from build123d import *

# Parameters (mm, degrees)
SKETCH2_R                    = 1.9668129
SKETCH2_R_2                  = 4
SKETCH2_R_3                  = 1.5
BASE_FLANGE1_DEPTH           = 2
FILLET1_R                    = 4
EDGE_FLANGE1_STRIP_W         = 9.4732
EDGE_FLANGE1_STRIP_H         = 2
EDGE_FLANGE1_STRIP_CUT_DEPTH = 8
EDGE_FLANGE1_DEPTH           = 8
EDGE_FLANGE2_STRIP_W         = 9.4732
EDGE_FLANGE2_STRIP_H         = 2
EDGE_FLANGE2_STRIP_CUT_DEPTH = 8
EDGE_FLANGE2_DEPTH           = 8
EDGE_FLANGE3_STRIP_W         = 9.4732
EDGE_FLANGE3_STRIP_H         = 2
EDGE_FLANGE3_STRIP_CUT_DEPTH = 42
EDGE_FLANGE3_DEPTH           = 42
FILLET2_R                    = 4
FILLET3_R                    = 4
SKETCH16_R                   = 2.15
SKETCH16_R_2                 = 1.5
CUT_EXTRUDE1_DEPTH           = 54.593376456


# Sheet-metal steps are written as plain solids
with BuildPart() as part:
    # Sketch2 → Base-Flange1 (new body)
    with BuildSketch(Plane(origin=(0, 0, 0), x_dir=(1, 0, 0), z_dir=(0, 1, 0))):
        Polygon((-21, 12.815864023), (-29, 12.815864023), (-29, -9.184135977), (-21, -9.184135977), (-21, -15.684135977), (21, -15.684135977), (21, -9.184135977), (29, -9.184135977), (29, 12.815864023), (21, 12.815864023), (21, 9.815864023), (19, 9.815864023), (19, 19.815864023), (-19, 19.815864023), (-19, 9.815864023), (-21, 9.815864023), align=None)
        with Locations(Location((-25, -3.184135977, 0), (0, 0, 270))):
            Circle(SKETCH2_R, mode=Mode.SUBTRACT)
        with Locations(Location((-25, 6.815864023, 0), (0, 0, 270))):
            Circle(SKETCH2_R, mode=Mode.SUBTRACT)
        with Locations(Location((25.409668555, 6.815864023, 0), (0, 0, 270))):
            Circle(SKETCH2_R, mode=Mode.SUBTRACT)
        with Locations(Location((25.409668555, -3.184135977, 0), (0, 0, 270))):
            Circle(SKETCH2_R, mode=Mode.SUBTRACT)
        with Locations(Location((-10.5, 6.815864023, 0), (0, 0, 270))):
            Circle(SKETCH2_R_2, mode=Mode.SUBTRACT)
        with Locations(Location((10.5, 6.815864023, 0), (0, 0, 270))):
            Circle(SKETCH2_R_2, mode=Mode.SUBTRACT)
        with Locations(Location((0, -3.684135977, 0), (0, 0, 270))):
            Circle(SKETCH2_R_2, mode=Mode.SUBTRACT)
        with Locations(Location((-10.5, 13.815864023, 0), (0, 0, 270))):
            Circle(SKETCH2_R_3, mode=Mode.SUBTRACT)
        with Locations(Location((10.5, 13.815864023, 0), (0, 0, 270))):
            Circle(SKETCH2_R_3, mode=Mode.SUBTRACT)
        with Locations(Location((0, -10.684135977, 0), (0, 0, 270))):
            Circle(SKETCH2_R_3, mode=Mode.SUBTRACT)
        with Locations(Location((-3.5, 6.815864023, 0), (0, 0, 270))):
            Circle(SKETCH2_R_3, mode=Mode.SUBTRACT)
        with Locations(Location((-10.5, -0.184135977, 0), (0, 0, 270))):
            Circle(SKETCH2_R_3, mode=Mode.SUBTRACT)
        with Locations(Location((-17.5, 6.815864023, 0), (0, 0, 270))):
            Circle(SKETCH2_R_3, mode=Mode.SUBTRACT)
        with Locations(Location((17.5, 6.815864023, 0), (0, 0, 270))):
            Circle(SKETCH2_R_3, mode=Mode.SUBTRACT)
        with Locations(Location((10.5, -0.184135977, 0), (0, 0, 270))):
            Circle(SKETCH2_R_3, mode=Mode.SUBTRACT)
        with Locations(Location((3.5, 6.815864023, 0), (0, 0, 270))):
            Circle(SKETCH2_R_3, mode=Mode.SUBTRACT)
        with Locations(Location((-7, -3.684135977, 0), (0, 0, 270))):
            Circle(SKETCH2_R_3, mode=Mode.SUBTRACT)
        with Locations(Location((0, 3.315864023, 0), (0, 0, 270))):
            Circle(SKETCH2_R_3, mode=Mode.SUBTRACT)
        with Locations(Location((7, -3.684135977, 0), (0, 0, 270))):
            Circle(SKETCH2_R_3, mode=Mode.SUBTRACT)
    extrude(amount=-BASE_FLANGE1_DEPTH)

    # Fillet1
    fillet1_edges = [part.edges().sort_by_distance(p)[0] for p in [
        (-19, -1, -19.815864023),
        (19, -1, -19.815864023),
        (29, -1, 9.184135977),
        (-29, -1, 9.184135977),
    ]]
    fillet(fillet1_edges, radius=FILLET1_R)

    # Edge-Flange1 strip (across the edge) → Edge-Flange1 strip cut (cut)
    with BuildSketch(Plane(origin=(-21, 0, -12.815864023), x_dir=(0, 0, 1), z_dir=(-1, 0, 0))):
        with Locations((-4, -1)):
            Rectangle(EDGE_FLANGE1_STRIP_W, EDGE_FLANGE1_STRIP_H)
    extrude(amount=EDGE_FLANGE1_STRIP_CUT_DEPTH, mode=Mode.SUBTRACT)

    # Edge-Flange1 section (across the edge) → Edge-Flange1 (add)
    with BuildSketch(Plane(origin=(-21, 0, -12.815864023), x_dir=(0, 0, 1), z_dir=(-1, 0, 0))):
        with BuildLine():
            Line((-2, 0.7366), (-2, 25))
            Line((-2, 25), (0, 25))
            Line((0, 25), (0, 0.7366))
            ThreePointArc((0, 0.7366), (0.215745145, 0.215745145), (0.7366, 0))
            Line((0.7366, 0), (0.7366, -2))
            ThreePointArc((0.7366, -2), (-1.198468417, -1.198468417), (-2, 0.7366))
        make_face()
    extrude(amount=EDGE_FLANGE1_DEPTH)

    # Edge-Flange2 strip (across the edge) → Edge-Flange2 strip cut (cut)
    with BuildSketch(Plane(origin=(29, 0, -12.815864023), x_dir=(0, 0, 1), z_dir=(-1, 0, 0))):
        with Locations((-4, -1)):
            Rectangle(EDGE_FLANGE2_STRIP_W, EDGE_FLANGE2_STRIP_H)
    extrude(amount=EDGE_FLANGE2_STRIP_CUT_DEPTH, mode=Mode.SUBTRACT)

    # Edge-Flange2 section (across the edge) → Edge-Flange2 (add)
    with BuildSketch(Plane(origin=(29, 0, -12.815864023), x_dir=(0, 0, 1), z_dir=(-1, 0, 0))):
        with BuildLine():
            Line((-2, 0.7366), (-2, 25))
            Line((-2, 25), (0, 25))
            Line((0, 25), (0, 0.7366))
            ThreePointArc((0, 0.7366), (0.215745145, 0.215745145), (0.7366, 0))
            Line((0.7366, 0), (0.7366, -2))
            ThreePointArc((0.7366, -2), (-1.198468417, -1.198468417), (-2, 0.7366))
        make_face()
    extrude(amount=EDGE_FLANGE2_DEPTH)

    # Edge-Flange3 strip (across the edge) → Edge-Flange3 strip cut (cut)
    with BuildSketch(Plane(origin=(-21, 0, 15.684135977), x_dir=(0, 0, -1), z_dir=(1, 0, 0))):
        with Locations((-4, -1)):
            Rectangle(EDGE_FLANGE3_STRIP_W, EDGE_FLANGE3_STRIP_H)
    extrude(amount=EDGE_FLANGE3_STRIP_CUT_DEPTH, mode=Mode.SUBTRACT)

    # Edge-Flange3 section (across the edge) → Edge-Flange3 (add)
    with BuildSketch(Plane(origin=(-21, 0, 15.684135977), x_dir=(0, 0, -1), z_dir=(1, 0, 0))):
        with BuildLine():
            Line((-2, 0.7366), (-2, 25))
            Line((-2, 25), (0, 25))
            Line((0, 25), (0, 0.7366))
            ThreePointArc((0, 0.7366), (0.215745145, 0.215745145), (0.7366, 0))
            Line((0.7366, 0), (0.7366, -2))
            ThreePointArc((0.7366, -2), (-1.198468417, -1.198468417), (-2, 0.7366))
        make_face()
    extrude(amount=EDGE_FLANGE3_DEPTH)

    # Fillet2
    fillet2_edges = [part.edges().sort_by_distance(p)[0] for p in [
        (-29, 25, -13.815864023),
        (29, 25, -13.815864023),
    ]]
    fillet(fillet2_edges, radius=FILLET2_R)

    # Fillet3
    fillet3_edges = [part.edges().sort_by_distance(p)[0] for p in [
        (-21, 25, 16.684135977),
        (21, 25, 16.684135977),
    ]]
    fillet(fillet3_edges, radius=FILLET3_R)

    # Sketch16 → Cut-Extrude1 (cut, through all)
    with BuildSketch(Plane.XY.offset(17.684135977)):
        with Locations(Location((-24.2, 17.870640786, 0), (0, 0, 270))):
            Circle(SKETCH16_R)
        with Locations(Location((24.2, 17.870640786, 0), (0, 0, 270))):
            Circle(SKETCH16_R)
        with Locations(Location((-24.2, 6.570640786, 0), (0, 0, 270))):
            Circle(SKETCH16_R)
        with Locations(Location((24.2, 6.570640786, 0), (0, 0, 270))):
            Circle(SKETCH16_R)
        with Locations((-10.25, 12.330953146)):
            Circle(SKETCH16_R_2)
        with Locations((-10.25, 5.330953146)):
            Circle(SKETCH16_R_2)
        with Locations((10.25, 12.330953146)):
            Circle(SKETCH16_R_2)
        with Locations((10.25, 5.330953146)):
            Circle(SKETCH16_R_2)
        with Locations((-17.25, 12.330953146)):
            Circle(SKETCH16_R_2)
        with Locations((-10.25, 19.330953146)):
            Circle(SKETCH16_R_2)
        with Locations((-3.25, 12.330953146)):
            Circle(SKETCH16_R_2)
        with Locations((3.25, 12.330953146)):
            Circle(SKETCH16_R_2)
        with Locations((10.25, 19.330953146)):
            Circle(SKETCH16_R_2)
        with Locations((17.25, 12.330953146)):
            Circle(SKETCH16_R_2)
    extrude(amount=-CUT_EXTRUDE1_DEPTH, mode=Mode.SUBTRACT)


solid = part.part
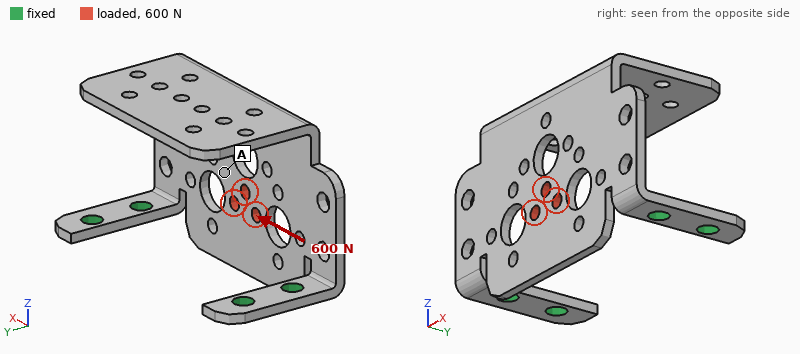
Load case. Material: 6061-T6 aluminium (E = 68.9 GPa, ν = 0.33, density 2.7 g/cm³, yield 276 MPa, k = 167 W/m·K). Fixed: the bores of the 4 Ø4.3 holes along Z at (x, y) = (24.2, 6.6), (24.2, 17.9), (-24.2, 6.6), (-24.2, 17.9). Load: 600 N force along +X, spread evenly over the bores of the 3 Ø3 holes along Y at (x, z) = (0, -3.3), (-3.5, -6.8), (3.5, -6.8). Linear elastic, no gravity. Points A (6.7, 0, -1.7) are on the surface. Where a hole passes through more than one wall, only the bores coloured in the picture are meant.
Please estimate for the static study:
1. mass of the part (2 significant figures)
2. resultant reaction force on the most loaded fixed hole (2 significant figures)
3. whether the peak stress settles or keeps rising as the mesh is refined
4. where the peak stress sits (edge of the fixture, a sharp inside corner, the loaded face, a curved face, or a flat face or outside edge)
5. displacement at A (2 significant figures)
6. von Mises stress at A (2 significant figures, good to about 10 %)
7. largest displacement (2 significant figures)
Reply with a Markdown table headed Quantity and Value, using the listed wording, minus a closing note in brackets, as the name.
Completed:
| Quantity | Value |
|---|---|
| mass of the part | 16 g |
| resultant reaction force on the most loaded fixed hole | 340 N |
| whether the peak stress settles or keeps rising as the mesh is refined | keeps rising |
| where the peak stress sits | edge of the fixture |
| displacement at A | 44 µm |
| von Mises stress at A | 21 MPa |
| largest displacement | 90 µm |
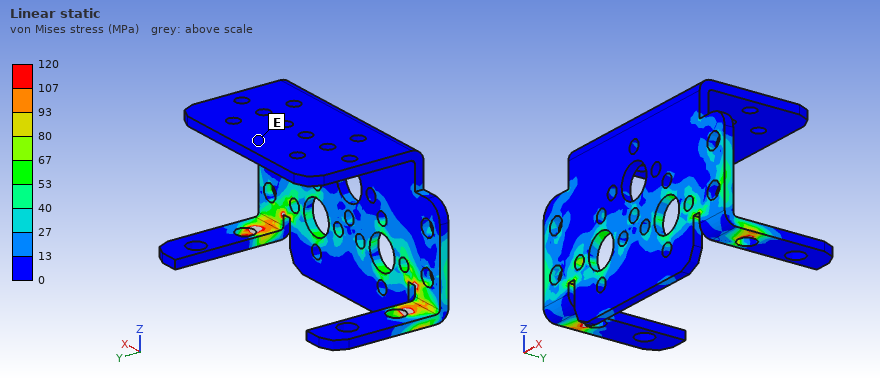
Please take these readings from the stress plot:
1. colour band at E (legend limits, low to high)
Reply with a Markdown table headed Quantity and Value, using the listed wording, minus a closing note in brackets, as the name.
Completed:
| Quantity | Value |
|---|---|
| colour band at E | 0 to 13 MPa |
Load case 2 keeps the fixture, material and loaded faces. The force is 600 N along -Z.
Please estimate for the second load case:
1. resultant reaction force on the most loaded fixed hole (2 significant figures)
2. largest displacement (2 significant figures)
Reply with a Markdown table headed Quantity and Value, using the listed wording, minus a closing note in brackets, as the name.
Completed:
| Quantity | Value |
|---|---|
| resultant reaction force on the most loaded fixed hole | 310 N |
| largest displacement | 0.54 mm |
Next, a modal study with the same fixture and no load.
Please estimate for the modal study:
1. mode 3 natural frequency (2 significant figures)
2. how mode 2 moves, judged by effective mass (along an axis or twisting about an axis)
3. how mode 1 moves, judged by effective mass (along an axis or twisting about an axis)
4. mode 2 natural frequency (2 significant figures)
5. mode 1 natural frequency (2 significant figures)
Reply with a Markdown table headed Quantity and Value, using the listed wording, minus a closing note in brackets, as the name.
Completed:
| Quantity | Value |
|---|---|
| mode 3 natural frequency | 1500 Hz |
| how mode 2 moves, judged by effective mass | along X |
| how mode 1 moves, judged by effective mass | along Y |
| mode 2 natural frequency | 1200 Hz |
| mode 1 natural frequency | 390 Hz |
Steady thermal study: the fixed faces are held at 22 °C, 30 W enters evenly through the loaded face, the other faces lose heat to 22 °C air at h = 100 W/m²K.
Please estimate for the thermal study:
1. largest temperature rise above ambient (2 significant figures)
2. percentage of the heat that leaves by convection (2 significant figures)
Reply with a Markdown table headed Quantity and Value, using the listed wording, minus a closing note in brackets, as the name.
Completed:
| Quantity | Value |
|---|---|
| largest temperature rise above ambient | 81 K |
| percentage of the heat that leaves by convection | 68 % |
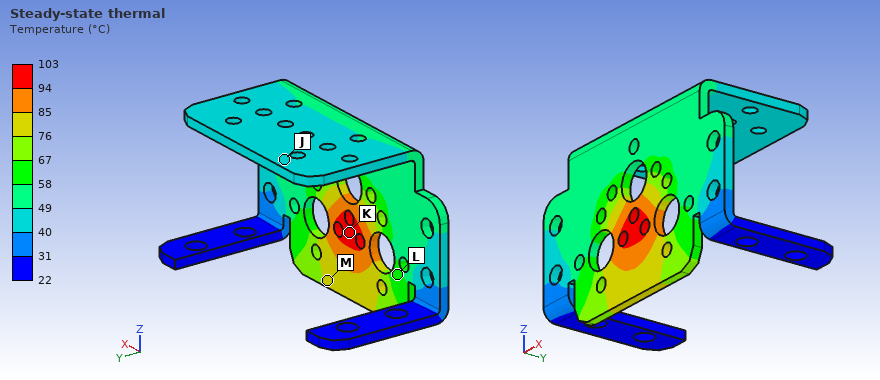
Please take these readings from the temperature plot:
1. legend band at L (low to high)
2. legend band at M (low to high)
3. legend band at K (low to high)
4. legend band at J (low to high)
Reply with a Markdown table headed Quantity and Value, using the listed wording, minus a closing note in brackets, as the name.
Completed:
| Quantity | Value |
|---|---|
| legend band at L | 58 to 67 °C |
| legend band at M | 76 to 85 °C |
| legend band at K | 94 to 103 °C |
| legend band at J | 40 to 49 °C |
